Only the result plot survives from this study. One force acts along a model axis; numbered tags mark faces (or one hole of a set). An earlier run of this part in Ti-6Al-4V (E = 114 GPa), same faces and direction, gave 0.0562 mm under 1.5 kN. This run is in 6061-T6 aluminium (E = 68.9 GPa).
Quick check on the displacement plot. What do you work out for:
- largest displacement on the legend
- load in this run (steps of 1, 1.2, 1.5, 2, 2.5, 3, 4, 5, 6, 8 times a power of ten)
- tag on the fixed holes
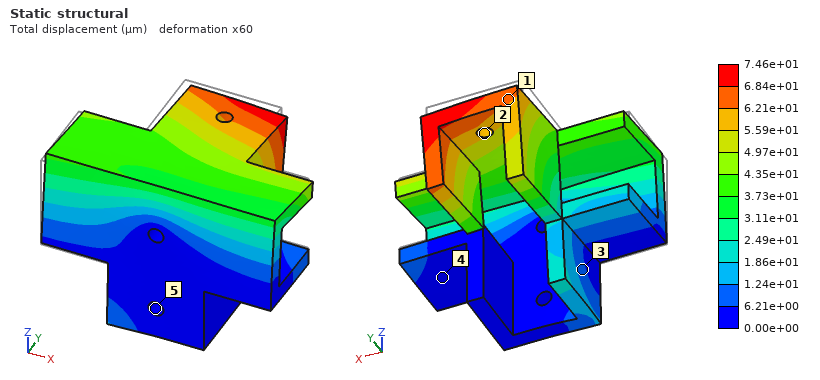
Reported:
7.46e+01 µm
1.2 kN
5
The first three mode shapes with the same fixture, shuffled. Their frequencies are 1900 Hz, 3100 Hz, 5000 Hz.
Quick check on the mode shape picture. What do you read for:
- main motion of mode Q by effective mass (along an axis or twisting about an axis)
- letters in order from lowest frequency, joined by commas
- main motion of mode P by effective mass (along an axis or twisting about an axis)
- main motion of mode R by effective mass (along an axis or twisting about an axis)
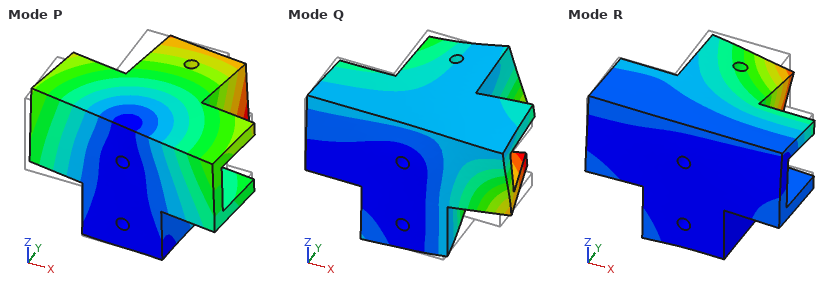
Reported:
along Y
P, R, Q
along X
along Z
